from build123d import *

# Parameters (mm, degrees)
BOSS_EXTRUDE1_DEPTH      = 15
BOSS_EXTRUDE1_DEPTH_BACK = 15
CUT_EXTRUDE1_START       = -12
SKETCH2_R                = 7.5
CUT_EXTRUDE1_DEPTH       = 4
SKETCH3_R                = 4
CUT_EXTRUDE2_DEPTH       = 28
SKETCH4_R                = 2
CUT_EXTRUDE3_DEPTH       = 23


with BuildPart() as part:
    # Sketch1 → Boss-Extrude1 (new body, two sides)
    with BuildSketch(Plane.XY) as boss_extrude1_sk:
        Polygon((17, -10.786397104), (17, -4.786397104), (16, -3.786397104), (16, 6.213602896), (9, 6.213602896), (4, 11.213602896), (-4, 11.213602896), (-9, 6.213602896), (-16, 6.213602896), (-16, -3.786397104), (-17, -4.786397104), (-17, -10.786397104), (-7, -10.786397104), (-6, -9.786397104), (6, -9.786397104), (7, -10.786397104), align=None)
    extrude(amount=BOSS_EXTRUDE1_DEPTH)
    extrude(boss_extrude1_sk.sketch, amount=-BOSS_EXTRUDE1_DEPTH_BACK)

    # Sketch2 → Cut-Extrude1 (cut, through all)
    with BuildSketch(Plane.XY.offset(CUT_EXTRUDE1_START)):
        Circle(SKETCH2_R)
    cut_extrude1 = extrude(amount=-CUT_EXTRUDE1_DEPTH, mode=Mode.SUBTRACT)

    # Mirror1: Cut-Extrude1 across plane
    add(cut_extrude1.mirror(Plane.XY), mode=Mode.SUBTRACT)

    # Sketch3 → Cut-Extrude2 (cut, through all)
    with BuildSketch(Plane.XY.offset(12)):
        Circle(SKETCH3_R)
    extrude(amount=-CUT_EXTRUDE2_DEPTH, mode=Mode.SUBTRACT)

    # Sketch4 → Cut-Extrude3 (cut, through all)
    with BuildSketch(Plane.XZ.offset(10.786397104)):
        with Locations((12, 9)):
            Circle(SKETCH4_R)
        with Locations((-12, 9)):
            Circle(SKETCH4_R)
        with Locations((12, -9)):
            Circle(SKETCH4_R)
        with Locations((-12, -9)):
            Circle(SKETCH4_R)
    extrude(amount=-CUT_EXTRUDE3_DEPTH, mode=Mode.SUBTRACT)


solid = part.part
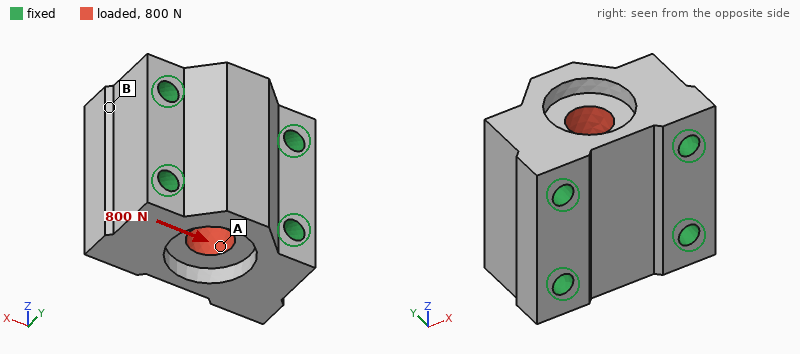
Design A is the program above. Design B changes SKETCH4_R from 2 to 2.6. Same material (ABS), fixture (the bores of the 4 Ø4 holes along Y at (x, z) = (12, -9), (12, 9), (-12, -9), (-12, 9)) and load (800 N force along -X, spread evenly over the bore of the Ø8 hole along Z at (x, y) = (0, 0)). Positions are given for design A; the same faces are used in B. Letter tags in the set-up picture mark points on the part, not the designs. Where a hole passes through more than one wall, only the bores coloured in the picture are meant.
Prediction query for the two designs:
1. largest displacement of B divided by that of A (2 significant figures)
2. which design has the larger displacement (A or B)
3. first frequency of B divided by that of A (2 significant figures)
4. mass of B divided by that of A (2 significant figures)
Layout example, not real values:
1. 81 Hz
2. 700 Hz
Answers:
1. 0.90
2. A
3. 1.1
4. 0.96
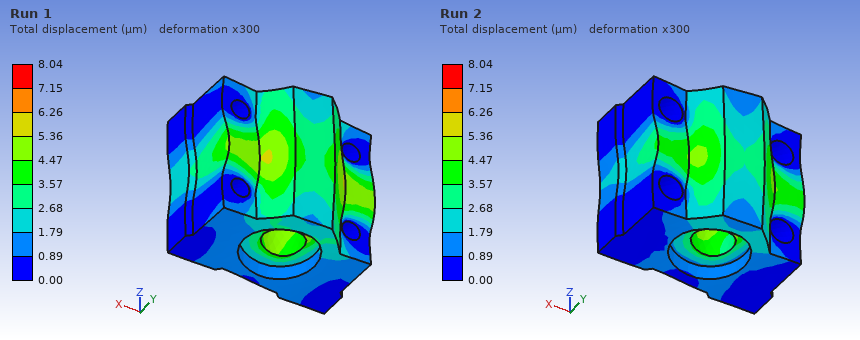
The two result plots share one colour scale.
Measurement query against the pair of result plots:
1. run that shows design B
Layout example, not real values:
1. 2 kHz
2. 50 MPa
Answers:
1. Run 2
